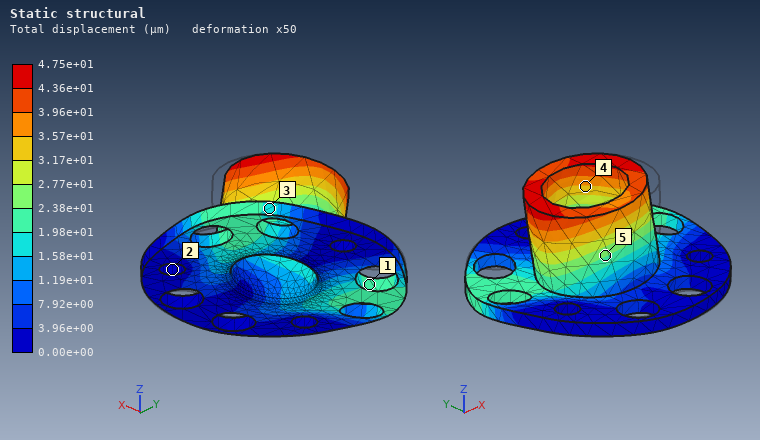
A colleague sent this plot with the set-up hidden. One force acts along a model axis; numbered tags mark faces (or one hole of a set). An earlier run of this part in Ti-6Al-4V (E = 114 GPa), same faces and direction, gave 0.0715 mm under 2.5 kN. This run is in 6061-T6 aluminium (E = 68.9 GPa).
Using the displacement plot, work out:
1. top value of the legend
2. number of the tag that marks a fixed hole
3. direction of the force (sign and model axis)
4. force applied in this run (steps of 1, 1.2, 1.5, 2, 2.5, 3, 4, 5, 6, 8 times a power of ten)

4.75e+01 µm
2
-X
1 kN
